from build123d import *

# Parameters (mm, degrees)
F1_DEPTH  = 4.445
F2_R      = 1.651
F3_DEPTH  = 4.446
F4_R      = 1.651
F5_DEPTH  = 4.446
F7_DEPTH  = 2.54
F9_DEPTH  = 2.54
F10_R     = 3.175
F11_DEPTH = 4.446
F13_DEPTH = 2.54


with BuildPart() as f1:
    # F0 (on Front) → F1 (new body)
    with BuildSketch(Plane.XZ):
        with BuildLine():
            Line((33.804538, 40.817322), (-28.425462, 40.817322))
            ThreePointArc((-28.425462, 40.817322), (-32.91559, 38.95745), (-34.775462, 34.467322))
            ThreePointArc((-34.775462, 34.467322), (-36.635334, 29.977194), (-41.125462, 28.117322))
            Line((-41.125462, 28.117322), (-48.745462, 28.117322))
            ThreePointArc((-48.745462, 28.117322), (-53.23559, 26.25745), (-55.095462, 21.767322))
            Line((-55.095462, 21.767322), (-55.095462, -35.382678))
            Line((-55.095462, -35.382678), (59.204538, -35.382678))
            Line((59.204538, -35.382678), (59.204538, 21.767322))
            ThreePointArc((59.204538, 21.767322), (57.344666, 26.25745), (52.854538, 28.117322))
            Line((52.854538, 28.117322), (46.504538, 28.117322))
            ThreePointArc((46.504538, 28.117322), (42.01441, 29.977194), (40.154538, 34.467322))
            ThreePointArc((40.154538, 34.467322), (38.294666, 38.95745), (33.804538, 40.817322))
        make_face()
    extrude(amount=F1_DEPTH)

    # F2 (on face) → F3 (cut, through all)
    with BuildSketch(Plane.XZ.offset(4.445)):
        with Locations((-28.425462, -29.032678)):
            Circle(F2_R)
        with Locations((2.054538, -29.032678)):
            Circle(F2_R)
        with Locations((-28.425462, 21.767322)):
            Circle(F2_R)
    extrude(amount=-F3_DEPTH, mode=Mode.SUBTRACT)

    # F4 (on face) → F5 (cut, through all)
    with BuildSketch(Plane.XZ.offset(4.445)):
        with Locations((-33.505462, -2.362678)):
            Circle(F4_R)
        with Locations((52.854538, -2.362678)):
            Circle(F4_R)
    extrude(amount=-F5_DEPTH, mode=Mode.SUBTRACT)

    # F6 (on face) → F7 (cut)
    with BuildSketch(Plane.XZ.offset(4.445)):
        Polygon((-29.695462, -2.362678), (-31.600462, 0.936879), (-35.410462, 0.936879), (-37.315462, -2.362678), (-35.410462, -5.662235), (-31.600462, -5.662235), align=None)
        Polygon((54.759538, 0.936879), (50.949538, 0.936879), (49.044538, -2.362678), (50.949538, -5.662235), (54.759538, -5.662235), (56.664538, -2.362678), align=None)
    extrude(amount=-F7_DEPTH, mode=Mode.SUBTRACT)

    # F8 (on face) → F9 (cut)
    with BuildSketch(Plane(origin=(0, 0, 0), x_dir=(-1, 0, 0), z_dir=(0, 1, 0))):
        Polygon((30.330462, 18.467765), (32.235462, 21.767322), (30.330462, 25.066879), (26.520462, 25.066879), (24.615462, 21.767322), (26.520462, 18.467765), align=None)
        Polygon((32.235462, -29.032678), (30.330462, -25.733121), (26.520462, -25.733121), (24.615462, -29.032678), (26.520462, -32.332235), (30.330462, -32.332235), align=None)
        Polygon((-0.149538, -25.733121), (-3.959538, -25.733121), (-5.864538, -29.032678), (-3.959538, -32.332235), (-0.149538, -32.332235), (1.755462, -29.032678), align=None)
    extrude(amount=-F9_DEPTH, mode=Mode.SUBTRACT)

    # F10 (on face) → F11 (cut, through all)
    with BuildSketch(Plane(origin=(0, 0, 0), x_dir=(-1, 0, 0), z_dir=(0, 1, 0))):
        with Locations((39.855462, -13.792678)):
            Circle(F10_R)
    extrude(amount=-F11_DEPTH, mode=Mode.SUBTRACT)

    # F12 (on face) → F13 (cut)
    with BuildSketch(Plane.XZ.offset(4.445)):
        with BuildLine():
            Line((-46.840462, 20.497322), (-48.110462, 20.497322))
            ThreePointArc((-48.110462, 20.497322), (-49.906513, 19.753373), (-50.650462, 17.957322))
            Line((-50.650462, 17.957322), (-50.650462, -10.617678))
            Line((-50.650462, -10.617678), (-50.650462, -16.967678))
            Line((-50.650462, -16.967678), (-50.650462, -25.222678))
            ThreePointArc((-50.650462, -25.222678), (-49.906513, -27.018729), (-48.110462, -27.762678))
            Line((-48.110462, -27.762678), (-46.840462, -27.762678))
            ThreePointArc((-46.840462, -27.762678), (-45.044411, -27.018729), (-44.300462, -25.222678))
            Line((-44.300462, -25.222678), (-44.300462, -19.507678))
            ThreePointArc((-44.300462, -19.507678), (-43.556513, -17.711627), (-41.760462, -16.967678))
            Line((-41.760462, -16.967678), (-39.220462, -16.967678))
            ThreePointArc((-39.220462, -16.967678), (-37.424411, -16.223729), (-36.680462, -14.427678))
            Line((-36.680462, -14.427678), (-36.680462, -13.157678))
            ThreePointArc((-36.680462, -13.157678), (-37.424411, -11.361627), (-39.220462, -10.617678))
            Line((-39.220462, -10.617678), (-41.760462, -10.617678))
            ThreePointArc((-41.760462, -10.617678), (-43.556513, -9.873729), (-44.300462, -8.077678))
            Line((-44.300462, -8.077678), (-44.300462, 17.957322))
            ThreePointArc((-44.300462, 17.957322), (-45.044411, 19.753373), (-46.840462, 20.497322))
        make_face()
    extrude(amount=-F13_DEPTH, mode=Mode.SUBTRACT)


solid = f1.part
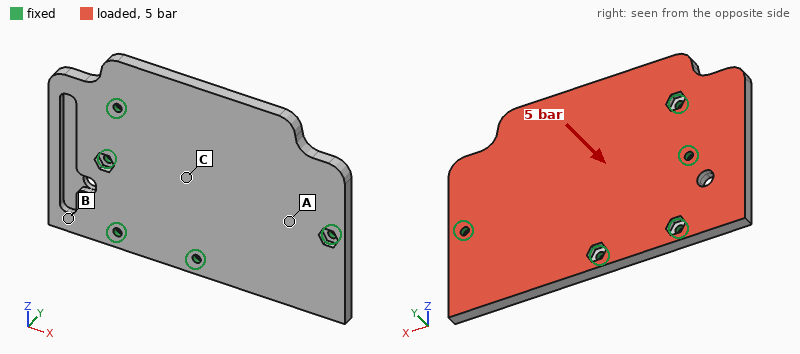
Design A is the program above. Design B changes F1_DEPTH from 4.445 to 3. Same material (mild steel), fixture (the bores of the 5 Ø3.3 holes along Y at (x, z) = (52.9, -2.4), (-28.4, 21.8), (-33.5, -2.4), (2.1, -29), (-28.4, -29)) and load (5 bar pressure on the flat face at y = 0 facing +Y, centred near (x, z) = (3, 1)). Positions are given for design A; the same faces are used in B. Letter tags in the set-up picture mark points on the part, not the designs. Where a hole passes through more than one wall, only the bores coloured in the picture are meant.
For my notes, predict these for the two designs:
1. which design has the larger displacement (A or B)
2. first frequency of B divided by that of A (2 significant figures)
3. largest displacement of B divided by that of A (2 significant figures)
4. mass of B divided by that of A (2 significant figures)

B
0.72
3.0
0.68
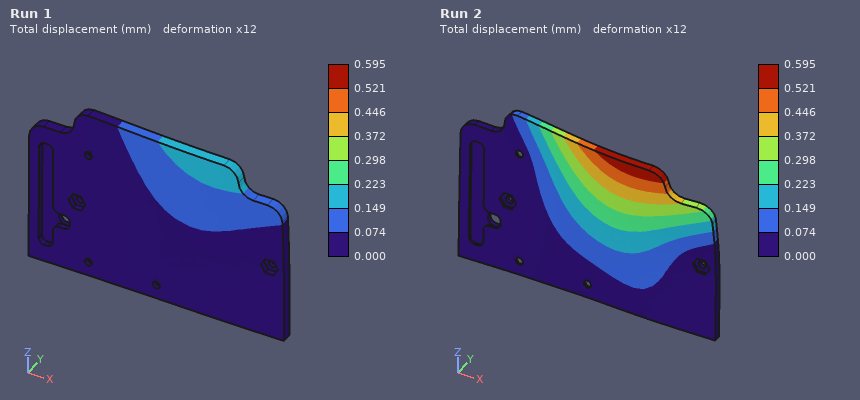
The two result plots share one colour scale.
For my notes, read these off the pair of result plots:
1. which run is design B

Run 2
